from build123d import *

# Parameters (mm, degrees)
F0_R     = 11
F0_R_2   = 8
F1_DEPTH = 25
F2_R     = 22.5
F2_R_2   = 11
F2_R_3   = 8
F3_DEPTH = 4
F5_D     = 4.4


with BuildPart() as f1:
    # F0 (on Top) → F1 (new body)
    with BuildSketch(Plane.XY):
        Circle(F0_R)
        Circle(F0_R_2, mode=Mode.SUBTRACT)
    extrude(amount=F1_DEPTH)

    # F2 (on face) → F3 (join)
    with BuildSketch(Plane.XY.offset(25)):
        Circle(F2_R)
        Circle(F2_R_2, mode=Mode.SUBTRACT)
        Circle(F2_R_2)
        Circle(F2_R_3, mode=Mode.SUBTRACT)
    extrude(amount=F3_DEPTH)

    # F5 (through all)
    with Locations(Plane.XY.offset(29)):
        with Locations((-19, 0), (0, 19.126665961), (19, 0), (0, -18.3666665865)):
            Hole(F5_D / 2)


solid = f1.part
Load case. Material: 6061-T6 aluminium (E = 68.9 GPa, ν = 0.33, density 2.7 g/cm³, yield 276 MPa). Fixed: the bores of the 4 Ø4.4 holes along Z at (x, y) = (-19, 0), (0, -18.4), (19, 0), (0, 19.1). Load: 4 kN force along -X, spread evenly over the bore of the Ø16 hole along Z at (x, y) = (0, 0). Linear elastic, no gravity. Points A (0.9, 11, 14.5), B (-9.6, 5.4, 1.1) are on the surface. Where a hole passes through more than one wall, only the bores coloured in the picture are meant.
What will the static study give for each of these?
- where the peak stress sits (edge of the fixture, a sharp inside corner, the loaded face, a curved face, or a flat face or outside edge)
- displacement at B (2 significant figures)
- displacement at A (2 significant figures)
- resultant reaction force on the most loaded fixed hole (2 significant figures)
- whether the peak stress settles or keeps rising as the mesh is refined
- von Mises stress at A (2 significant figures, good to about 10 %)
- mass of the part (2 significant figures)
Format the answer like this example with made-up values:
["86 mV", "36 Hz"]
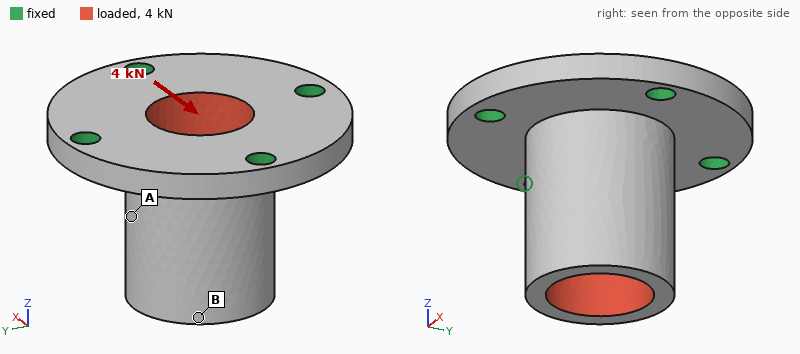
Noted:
["edge of the fixture", "93 µm", "43 µm", "2.0 kN", "keeps rising", "33 MPa", "26 g"]
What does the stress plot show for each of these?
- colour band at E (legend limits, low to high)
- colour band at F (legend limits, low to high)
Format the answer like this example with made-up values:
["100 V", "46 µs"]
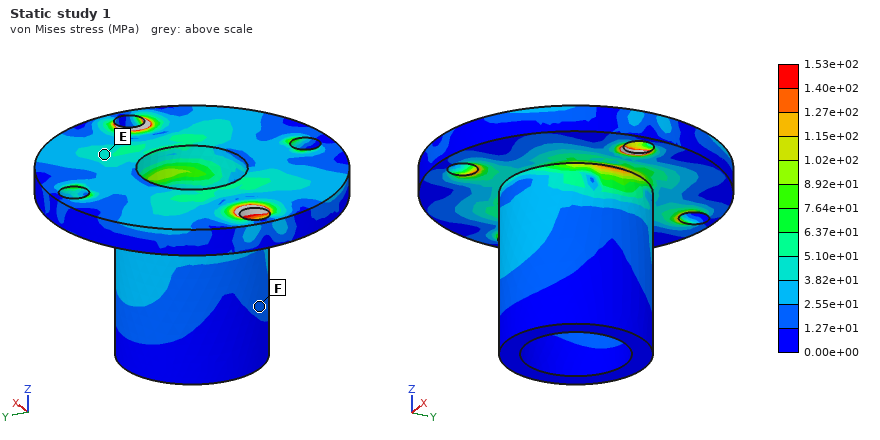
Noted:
["3.82e+01 to 5.10e+01 MPa", "1.27e+01 to 2.55e+01 MPa"]
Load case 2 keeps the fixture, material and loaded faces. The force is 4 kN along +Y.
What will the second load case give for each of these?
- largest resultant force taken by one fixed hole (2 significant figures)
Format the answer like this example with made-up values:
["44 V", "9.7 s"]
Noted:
["2.1 kN"]
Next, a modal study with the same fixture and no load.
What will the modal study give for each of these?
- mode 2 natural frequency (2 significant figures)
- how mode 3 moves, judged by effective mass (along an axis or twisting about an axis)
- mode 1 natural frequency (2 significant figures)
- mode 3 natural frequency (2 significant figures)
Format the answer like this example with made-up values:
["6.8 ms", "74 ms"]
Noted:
["10000 Hz", "along Z", "9900 Hz", "17 kHz"]
